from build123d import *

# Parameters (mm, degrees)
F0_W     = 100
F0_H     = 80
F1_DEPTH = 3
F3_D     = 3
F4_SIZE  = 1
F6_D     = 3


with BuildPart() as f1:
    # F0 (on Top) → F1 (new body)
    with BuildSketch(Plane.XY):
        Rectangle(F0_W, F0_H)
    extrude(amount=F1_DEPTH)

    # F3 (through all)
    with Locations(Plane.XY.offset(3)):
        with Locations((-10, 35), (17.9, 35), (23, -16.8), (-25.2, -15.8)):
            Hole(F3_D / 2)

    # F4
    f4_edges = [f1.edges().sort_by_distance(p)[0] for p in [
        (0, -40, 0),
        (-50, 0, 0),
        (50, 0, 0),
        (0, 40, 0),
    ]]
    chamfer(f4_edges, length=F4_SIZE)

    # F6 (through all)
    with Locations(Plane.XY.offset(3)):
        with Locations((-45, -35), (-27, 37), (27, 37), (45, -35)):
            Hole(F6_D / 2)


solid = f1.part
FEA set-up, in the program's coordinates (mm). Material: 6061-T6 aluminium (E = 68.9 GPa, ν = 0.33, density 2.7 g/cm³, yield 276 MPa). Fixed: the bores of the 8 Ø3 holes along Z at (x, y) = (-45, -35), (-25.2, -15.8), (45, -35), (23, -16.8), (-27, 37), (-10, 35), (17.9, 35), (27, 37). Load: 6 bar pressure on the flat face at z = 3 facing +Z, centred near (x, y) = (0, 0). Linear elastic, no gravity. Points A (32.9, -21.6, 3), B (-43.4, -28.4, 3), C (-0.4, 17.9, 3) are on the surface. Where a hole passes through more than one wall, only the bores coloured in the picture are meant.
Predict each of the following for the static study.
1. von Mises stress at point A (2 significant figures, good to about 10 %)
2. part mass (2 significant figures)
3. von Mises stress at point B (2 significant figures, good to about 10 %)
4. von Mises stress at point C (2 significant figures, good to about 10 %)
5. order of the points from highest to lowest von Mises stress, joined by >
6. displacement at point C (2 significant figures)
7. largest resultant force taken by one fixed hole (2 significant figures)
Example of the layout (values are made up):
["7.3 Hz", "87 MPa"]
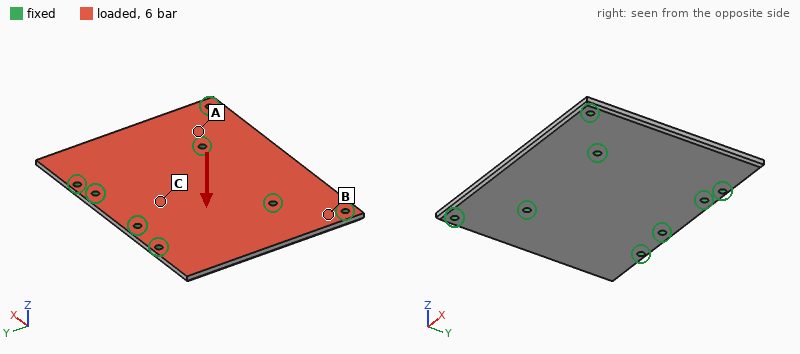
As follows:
["75 MPa", "64 g", "53 MPa", "23 MPa", "A > B > C", "0.074 mm", "1.2 kN"]
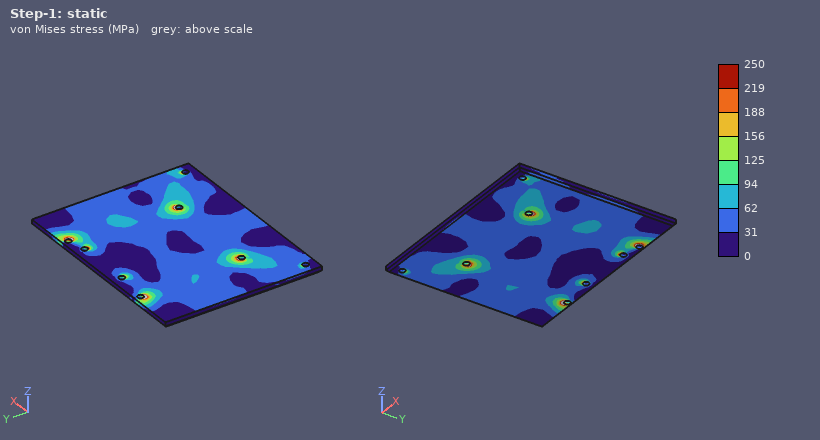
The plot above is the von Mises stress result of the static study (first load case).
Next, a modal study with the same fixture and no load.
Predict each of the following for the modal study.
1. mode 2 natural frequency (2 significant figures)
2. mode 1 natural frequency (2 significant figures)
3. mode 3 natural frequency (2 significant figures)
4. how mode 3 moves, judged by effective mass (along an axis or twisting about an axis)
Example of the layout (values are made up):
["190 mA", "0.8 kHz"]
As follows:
["3300 Hz", "3200 Hz", "4100 Hz", "along Z"]
